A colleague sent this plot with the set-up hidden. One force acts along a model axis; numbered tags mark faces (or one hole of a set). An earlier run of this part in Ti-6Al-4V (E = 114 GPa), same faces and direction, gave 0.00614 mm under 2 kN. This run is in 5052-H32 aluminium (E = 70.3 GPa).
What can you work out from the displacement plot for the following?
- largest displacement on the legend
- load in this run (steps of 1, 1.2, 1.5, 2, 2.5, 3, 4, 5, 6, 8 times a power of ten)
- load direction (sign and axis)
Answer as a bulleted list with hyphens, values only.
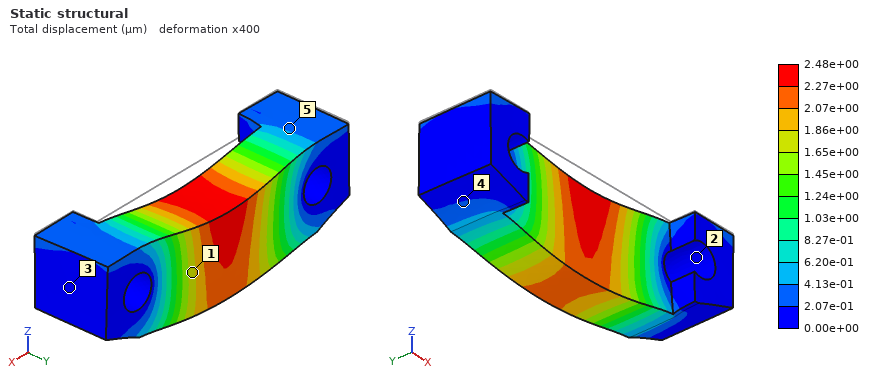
- 2.48e+00 µm
- 500 N
- -Z
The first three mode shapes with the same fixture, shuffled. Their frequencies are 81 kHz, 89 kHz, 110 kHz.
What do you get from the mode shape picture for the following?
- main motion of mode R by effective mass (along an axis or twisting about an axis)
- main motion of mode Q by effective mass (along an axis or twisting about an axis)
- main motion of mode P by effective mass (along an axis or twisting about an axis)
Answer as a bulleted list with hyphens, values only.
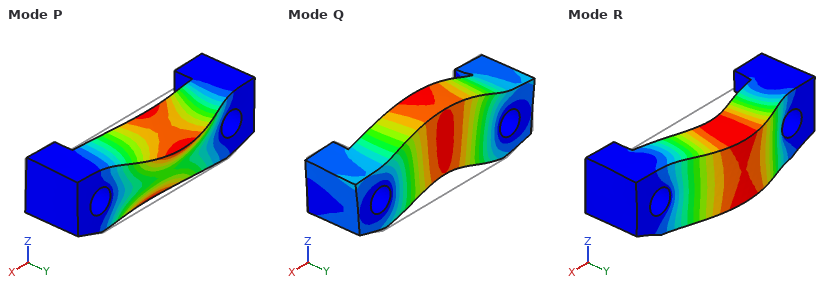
- along Y
- along Z
- twisting about X
